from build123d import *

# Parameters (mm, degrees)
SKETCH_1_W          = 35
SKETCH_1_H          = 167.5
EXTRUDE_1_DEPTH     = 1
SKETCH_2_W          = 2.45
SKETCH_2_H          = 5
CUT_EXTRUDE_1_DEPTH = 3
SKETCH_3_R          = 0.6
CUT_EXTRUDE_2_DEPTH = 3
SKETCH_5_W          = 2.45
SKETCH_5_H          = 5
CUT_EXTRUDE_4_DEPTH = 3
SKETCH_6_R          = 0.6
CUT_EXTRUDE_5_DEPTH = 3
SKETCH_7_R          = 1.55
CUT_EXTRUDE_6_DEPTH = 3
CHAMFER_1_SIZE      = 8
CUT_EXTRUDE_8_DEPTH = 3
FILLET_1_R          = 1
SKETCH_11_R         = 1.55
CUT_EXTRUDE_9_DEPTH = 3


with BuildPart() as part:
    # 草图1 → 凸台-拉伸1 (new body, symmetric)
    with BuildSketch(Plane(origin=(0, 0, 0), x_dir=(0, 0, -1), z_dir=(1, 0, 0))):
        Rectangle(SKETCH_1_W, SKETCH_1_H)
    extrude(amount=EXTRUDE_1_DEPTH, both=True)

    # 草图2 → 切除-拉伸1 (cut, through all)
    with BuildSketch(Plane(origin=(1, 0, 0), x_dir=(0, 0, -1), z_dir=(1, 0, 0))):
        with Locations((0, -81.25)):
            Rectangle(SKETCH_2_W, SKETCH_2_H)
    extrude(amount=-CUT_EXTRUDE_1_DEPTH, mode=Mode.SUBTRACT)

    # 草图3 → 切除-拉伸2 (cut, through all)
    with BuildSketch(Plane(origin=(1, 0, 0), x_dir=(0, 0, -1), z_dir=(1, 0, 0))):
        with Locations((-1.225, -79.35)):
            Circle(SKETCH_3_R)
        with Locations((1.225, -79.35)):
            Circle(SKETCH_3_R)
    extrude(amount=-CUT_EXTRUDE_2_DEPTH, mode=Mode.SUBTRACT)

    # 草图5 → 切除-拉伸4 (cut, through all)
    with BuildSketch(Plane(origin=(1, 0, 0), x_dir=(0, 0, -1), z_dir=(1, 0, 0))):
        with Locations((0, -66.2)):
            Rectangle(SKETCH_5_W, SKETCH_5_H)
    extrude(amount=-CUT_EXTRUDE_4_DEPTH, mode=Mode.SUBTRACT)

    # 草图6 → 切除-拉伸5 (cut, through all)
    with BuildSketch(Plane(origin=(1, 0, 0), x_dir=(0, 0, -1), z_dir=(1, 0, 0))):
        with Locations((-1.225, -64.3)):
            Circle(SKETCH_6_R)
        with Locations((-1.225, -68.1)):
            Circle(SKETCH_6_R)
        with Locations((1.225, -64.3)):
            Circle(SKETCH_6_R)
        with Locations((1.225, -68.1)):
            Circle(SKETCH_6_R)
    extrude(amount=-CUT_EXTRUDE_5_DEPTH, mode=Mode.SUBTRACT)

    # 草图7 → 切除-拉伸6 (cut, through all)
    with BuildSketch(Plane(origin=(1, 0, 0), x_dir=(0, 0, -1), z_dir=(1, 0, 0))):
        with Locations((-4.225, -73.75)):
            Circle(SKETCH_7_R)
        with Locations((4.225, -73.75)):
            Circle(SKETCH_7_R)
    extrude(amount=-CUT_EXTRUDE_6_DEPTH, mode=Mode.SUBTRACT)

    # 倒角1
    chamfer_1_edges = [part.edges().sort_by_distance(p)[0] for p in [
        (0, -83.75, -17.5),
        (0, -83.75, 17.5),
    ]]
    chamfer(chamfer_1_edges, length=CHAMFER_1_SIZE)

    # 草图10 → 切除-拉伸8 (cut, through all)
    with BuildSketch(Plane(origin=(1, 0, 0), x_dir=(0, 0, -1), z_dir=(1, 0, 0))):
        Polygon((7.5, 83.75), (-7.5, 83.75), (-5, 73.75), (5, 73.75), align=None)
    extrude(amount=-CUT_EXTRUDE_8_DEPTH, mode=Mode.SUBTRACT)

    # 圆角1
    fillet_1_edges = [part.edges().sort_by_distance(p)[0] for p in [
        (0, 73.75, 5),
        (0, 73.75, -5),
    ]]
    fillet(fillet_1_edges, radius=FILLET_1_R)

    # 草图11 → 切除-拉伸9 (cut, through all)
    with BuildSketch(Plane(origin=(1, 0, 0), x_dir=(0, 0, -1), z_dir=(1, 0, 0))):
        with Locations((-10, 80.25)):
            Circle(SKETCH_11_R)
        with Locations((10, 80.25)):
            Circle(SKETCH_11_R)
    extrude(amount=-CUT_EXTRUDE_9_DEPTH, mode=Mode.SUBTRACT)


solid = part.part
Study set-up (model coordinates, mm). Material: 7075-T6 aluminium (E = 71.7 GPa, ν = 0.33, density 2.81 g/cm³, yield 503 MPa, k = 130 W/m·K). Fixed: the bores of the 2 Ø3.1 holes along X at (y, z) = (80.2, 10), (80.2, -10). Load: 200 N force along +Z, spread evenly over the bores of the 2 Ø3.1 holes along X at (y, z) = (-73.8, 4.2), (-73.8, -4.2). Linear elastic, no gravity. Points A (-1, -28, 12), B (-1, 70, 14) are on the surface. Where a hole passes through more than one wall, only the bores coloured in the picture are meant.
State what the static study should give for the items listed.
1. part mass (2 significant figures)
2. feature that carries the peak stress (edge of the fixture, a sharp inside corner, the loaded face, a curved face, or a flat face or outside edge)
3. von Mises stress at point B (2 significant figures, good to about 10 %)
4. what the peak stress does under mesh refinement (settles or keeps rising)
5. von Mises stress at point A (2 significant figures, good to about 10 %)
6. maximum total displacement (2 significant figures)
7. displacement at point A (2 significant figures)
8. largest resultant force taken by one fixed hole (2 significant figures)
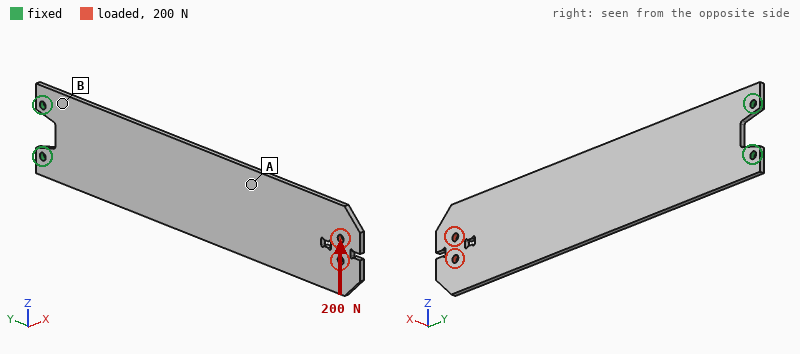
32 g
edge of the fixture
53 MPa
keeps rising
16 MPa
0.62 mm
0.34 mm
1.4 kN
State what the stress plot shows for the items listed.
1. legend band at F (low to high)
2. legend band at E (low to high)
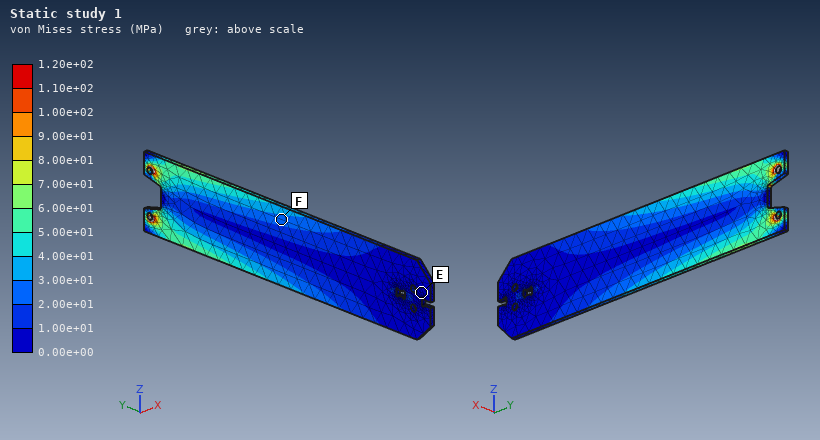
2.00e+01 to 3.00e+01 MPa
0.00e+00 to 1.00e+01 MPa
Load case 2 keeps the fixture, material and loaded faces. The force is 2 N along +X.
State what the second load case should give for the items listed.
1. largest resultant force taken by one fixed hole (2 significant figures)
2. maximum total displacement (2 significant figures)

1.0 N
1.7 mm
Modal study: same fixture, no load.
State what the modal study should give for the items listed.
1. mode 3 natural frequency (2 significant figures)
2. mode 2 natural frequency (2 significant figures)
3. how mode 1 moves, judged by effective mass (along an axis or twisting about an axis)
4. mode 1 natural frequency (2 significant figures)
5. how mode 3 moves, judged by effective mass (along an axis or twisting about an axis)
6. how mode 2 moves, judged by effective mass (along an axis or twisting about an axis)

570 Hz
380 Hz
along X
61 Hz
twisting about Y
along X
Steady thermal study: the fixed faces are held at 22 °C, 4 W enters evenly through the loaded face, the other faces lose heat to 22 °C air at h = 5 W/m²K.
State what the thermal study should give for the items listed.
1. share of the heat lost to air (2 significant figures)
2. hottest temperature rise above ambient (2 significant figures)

38 %
53 K
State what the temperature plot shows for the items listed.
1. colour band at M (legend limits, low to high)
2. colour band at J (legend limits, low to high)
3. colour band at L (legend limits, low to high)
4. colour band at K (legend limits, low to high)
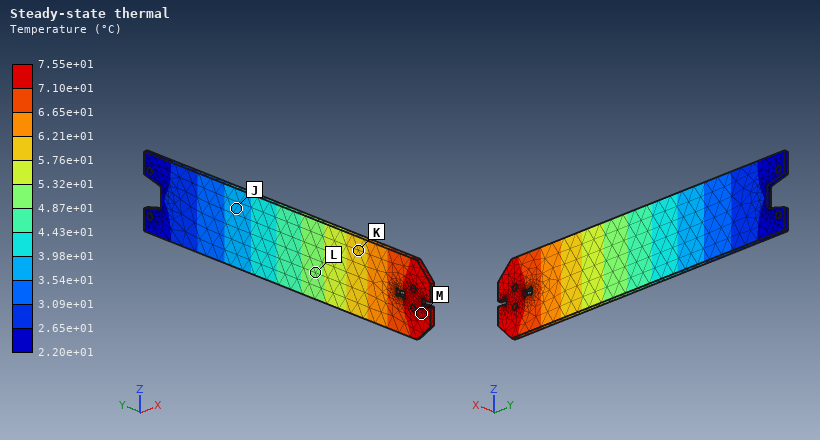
7.10e+01 to 7.55e+01 °C
3.54e+01 to 3.98e+01 °C
4.87e+01 to 5.32e+01 °C
5.76e+01 to 6.21e+01 °C
